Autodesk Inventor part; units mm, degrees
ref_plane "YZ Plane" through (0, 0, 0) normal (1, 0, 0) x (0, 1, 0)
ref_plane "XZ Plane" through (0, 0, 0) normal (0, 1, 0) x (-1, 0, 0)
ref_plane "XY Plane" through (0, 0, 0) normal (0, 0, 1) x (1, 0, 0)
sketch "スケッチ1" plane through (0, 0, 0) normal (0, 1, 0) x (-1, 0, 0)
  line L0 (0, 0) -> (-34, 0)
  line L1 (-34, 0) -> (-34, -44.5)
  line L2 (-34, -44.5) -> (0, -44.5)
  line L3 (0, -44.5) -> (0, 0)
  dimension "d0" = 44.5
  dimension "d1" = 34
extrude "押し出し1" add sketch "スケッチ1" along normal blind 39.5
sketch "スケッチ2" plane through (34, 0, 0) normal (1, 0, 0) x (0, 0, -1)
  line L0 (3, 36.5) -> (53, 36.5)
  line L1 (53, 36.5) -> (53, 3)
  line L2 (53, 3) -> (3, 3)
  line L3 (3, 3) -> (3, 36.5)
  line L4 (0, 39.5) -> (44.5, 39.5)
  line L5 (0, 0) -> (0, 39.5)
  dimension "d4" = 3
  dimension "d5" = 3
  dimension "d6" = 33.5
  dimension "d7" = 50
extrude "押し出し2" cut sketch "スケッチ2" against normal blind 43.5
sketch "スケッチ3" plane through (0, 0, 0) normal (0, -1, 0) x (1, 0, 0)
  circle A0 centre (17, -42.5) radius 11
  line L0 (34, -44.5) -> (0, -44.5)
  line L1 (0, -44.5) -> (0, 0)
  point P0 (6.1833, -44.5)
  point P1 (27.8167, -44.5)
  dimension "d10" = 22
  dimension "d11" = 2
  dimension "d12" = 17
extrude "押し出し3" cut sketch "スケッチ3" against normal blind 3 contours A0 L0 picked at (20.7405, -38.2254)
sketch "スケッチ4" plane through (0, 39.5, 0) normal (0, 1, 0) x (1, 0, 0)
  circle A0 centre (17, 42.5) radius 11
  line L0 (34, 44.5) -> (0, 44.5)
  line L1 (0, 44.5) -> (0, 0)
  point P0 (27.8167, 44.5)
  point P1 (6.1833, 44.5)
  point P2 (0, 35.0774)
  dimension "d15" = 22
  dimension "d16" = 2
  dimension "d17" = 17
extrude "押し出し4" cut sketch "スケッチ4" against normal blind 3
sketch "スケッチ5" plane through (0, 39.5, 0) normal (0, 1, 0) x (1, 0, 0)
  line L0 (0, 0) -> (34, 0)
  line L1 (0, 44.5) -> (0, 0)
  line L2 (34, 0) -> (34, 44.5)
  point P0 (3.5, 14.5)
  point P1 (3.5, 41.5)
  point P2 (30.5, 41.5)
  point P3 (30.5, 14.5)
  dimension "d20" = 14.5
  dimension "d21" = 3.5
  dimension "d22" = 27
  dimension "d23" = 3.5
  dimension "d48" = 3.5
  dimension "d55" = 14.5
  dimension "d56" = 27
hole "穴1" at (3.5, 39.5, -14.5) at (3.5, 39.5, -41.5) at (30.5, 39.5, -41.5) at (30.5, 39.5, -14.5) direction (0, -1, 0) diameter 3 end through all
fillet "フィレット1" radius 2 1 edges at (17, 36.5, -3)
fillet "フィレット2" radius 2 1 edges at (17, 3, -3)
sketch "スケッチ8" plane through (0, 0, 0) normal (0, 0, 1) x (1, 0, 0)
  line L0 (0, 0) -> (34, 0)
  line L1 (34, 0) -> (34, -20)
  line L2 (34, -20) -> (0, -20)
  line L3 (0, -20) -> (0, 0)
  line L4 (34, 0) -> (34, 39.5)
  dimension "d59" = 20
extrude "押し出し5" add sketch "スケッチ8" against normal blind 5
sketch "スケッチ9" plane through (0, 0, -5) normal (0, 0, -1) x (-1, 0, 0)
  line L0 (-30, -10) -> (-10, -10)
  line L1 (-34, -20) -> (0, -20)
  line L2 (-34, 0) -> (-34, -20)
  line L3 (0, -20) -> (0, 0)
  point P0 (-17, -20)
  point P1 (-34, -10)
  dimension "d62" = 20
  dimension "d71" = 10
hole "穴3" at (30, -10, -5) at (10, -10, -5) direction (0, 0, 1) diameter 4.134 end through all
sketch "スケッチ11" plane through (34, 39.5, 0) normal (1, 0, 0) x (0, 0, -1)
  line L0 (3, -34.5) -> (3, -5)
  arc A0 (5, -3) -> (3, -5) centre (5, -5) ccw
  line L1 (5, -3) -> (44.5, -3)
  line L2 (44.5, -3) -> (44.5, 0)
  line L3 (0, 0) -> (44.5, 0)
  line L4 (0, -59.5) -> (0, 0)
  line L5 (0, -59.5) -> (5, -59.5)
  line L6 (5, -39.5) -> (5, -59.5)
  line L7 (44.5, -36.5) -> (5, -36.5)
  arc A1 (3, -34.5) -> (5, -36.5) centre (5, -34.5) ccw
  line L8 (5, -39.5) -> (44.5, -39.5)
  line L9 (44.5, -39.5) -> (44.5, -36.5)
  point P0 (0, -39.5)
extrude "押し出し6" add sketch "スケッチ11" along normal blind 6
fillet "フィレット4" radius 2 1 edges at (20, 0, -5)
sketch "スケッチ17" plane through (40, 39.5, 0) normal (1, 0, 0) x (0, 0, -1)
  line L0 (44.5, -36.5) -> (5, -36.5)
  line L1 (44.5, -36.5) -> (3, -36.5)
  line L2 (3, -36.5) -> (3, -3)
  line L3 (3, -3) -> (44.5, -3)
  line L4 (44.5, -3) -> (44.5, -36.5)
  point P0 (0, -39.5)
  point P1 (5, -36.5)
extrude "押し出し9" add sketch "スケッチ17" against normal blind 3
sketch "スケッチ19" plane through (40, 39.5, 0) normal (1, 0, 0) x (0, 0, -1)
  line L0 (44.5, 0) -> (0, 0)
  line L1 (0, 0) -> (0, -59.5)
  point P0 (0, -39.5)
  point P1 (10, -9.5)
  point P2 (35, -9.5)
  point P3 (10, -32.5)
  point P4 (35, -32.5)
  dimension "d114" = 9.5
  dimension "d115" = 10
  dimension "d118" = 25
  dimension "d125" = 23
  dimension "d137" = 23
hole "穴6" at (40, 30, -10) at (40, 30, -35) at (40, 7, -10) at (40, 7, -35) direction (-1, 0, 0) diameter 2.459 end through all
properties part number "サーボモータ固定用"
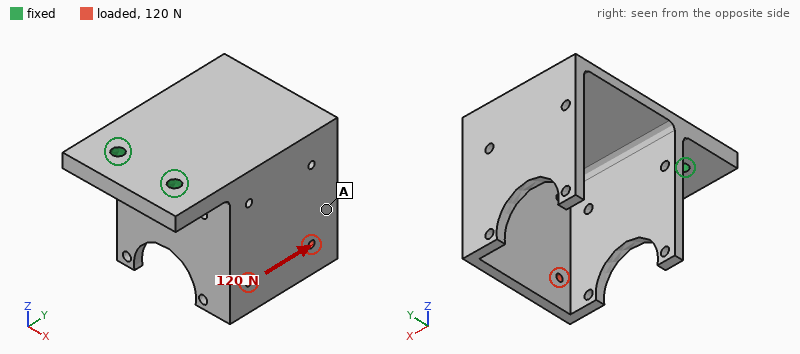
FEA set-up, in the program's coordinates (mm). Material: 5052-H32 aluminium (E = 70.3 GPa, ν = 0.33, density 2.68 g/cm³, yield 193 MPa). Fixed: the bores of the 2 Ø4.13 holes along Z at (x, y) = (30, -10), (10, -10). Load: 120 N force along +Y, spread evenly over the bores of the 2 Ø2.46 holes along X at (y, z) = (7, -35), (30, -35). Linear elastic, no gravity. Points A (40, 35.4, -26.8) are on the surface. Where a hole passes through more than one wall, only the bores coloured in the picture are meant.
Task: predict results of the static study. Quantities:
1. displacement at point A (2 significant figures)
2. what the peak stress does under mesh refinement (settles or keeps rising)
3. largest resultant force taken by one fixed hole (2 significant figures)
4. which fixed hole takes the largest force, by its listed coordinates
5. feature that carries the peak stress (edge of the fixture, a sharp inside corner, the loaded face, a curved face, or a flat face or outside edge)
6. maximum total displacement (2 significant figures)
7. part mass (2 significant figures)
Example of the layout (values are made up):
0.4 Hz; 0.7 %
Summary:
0.13 mm; keeps rising; 160 N; (30, -10); edge of the fixture; 0.18 mm; 57 g
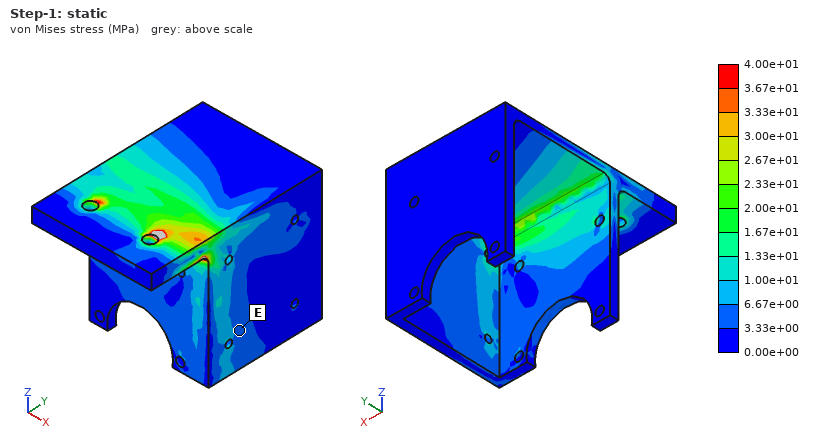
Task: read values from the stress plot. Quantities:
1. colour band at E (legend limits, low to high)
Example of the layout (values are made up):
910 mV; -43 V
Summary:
3.33e+00 to 6.67e+00 MPa
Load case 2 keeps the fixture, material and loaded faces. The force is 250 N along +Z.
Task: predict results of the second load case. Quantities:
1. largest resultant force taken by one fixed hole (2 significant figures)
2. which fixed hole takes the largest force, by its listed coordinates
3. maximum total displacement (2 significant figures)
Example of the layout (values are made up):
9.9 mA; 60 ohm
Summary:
310 N; (30, -10); 0.25 mm
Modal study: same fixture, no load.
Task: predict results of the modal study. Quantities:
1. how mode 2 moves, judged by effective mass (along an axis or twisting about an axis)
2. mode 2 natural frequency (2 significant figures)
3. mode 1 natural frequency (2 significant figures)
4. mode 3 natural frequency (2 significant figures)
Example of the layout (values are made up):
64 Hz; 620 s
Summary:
along X; 1500 Hz; 840 Hz; 2600 Hz
